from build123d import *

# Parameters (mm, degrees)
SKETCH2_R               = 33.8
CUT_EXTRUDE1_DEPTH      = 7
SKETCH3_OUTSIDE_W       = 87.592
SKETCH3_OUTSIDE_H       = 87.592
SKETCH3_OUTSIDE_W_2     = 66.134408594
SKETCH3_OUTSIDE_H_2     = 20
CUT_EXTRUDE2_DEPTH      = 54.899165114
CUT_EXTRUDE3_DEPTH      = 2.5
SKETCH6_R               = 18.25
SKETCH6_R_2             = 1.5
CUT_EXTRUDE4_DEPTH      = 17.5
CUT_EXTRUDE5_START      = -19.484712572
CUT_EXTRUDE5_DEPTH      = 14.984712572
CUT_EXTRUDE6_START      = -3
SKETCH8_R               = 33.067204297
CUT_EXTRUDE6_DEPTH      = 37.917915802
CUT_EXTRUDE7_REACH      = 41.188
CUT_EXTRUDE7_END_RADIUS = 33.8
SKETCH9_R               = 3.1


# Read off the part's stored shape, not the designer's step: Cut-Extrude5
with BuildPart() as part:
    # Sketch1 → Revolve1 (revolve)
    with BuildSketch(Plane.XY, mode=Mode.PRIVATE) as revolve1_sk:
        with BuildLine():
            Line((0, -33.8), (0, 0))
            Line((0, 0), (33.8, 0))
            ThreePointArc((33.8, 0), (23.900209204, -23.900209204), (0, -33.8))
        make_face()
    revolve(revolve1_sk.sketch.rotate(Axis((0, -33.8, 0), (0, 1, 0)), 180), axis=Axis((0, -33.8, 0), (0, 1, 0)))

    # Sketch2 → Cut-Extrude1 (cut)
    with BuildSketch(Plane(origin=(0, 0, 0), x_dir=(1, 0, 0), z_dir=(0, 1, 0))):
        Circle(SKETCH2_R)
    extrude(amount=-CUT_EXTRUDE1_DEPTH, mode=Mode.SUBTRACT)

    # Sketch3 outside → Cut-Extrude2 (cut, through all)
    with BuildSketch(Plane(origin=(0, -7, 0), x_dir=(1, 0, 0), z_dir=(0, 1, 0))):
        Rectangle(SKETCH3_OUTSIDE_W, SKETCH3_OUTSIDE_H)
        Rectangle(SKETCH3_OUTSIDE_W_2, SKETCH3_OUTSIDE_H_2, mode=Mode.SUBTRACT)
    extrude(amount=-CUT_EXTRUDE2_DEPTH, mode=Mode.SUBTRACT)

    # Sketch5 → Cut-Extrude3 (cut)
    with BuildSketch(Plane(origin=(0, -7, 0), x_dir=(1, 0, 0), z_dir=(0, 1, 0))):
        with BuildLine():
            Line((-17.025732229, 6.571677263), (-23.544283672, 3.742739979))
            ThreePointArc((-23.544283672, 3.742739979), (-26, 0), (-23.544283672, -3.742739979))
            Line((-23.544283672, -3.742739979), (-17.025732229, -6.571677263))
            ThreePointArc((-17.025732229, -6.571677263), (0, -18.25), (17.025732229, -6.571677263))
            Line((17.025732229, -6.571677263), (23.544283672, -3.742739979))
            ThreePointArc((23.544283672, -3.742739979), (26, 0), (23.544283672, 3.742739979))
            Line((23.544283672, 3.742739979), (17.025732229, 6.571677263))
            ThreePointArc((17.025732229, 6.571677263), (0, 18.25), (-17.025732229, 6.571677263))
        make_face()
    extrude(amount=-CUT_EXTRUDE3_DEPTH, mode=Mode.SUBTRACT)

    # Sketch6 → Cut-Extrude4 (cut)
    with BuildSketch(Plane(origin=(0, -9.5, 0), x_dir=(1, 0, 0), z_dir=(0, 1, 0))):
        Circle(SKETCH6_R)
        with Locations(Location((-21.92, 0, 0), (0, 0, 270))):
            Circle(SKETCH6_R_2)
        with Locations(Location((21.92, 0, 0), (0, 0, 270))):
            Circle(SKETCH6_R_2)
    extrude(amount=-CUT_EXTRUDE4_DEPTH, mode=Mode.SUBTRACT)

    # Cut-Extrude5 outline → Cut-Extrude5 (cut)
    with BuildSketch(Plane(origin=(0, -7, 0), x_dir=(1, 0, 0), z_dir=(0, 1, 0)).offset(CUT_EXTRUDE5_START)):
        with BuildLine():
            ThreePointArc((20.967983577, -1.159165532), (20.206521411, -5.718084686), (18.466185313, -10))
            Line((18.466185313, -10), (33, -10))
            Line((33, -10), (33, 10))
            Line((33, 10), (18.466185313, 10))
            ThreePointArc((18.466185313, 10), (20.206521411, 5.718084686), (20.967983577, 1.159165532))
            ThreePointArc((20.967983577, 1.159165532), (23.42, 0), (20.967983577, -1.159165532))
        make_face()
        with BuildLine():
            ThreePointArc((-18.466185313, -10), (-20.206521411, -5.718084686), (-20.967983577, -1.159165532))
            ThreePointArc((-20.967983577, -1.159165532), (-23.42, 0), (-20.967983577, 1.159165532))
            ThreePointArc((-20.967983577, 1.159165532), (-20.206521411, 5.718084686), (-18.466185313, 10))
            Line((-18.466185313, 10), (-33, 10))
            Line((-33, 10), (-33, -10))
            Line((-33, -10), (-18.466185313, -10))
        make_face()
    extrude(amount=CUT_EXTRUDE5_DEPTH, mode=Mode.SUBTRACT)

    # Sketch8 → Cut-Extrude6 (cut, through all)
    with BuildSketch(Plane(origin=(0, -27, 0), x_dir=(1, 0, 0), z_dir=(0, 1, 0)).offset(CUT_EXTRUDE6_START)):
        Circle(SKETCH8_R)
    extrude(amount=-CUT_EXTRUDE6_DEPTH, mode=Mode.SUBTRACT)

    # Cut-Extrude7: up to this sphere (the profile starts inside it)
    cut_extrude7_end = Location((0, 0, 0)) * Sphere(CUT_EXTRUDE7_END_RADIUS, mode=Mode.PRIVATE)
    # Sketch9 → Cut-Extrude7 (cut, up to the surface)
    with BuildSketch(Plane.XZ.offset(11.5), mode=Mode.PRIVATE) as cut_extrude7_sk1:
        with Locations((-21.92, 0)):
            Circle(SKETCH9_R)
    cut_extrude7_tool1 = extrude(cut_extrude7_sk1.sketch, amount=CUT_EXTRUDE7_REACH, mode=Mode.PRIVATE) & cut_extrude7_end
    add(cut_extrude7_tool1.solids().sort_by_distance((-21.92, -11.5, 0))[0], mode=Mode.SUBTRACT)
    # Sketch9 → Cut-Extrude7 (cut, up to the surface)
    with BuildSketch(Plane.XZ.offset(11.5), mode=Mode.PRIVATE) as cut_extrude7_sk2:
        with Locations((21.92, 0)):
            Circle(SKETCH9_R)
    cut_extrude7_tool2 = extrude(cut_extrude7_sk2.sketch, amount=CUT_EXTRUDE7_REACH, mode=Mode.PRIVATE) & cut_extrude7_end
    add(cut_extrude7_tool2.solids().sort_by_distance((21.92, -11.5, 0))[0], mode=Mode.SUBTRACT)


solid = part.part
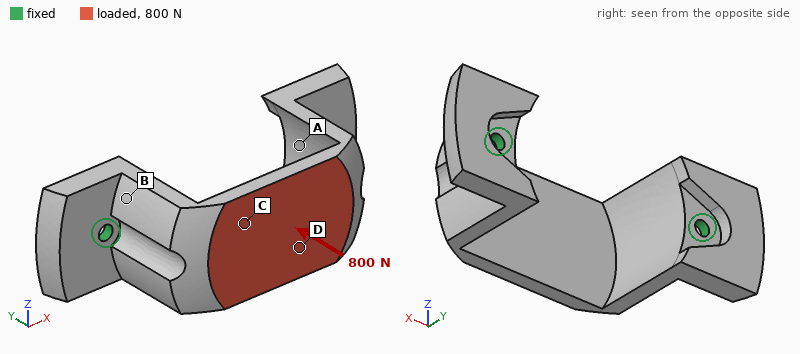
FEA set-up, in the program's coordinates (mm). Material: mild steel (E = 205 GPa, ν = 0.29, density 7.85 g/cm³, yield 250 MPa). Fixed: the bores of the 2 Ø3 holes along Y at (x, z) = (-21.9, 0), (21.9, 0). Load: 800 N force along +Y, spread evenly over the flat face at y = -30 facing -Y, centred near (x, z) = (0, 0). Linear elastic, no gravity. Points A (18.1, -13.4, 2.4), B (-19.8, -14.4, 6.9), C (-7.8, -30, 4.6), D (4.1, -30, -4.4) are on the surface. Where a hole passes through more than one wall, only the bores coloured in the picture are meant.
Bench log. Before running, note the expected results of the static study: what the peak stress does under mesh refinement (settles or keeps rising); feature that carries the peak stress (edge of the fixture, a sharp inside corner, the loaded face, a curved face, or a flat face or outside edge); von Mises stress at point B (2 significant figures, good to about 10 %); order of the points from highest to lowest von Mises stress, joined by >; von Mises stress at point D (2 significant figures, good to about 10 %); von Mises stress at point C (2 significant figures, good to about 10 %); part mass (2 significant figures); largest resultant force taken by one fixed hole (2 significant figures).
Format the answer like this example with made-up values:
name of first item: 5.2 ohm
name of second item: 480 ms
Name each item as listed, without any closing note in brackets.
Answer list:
what the peak stress does under mesh refinement: keeps rising
feature that carries the peak stress: a sharp inside corner
von Mises stress at point B: 23 MPa
order of the points from highest to lowest von Mises stress, joined by >: D > C > B > A
von Mises stress at point D: 78 MPa
von Mises stress at point C: 59 MPa
part mass: 46 g
largest resultant force taken by one fixed hole: 430 N
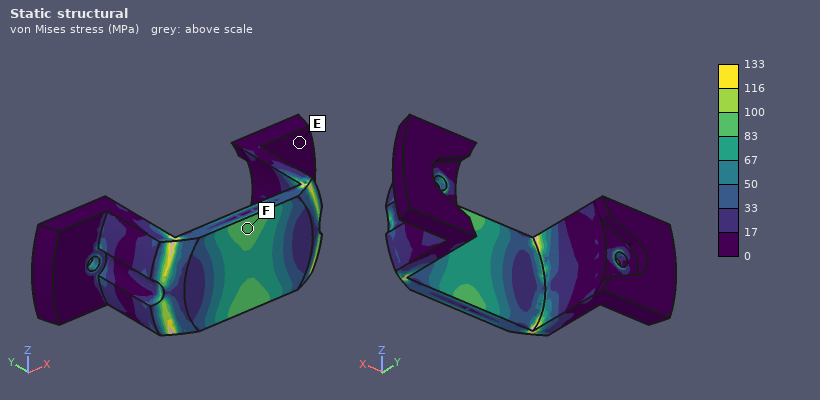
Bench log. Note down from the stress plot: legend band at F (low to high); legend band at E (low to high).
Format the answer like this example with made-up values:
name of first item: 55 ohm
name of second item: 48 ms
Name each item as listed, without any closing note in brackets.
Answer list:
legend band at F: 83 to 100 MPa
legend band at E: 0 to 17 MPa
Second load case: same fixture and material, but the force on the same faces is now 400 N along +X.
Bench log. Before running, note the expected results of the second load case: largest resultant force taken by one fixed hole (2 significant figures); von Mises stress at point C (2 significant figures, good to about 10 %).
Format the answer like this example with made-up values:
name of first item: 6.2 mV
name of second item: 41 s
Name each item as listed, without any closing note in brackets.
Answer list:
largest resultant force taken by one fixed hole: 220 N
von Mises stress at point C: 22 MPa
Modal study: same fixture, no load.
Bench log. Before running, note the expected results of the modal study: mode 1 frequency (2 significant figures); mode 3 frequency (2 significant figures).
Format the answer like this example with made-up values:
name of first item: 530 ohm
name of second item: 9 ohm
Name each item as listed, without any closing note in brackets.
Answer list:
mode 1 frequency: 3400 Hz
mode 3 frequency: 6100 Hz
